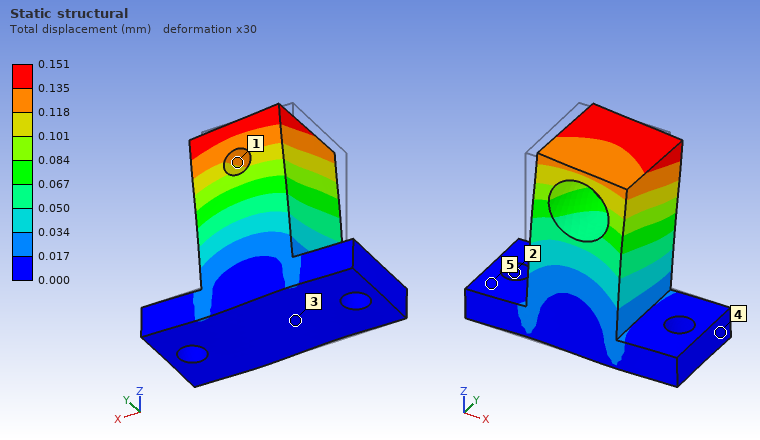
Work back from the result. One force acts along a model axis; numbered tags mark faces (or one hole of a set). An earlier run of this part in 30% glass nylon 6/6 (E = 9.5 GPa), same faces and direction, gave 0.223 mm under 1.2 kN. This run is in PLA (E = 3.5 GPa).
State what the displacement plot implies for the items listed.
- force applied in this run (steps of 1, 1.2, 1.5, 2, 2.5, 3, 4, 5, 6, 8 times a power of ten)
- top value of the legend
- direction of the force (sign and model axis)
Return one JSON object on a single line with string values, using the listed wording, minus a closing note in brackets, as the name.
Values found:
{"force applied in this run": "300 N", "top value of the legend": "0.151 mm", "direction of the force": "+X"}
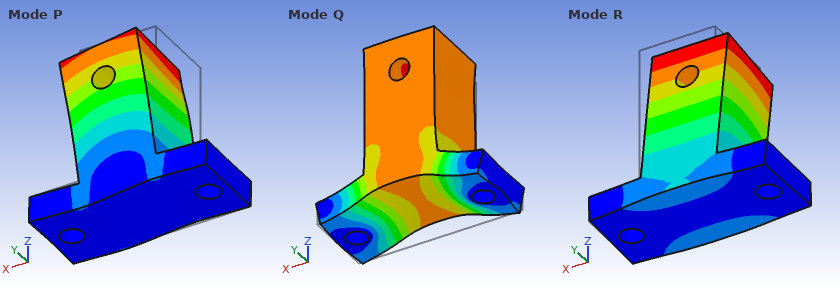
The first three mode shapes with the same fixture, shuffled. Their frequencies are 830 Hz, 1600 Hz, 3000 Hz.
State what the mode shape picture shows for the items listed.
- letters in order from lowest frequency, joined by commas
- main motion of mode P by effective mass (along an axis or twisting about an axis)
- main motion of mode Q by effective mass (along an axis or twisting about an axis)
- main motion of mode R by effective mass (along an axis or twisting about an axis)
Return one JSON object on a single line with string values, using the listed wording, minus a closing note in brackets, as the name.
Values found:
{"letters in order from lowest frequency, joined by commas": "R, P, Q", "main motion of mode P by effective mass": "along X", "main motion of mode Q by effective mass": "along Z", "main motion of mode R by effective mass": "along Y"}
